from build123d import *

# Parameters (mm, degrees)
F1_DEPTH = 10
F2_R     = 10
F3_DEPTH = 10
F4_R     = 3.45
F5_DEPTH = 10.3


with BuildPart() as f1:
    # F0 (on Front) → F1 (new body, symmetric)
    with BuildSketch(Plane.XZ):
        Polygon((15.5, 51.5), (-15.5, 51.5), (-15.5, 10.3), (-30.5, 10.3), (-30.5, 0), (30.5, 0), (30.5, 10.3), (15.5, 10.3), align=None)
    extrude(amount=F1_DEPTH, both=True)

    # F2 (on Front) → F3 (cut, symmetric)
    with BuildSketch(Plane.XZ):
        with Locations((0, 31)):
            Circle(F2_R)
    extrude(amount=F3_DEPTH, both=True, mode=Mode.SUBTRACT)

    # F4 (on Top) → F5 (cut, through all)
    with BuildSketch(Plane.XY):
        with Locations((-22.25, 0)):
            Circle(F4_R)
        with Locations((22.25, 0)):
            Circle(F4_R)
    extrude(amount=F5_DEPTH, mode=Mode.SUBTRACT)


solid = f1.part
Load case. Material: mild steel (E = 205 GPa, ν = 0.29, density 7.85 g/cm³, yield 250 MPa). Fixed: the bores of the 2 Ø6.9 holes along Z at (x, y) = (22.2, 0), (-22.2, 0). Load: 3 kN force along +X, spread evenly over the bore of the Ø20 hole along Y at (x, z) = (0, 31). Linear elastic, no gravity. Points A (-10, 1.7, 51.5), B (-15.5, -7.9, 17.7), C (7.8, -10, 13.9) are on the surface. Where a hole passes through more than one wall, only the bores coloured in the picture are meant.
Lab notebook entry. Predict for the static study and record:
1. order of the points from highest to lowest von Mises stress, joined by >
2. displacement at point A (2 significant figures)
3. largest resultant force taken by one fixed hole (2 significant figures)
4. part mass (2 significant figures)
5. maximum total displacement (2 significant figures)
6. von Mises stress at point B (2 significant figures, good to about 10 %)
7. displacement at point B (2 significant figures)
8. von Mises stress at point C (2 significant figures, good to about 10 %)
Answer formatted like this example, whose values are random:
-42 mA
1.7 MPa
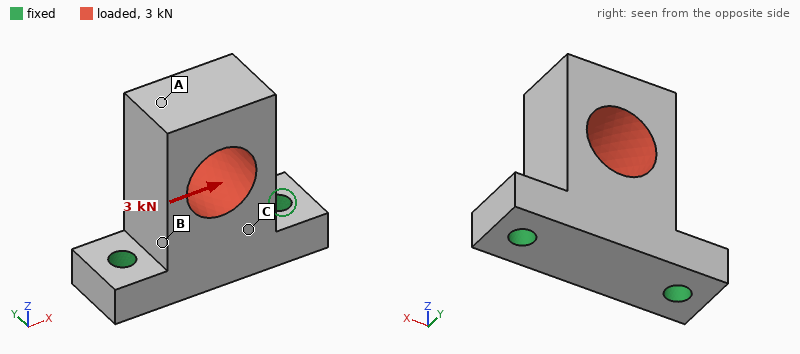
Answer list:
B > C > A
15 µm
2.6 kN
240 g
15 µm
26 MPa
3.2 µm
11 MPa
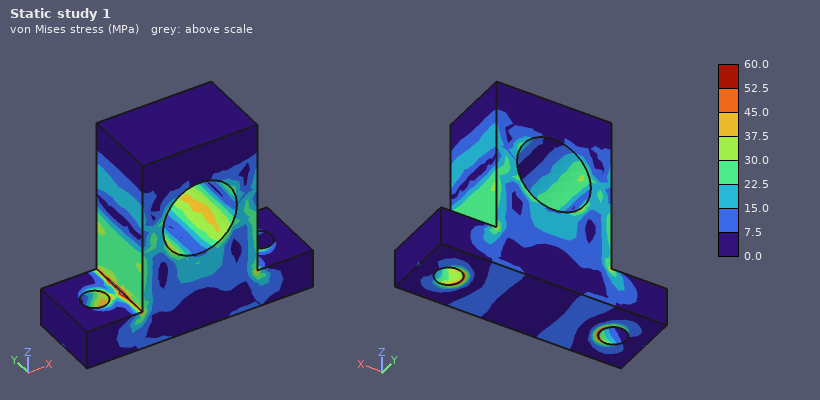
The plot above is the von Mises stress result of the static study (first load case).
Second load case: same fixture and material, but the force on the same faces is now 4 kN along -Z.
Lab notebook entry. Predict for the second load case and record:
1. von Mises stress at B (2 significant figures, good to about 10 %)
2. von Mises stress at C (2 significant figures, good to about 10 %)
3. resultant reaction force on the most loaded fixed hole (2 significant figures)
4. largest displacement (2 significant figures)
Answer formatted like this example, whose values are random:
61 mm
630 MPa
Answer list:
13 MPa
5.7 MPa
2.1 kN
3.7 µm
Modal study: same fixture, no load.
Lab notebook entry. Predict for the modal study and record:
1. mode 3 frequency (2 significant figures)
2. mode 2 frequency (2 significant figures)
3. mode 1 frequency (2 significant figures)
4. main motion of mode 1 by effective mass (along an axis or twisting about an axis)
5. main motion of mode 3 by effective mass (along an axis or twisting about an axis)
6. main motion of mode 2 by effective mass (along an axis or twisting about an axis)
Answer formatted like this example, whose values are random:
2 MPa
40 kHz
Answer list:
11 kHz
6400 Hz
3700 Hz
along Y
twisting about Z
along X
